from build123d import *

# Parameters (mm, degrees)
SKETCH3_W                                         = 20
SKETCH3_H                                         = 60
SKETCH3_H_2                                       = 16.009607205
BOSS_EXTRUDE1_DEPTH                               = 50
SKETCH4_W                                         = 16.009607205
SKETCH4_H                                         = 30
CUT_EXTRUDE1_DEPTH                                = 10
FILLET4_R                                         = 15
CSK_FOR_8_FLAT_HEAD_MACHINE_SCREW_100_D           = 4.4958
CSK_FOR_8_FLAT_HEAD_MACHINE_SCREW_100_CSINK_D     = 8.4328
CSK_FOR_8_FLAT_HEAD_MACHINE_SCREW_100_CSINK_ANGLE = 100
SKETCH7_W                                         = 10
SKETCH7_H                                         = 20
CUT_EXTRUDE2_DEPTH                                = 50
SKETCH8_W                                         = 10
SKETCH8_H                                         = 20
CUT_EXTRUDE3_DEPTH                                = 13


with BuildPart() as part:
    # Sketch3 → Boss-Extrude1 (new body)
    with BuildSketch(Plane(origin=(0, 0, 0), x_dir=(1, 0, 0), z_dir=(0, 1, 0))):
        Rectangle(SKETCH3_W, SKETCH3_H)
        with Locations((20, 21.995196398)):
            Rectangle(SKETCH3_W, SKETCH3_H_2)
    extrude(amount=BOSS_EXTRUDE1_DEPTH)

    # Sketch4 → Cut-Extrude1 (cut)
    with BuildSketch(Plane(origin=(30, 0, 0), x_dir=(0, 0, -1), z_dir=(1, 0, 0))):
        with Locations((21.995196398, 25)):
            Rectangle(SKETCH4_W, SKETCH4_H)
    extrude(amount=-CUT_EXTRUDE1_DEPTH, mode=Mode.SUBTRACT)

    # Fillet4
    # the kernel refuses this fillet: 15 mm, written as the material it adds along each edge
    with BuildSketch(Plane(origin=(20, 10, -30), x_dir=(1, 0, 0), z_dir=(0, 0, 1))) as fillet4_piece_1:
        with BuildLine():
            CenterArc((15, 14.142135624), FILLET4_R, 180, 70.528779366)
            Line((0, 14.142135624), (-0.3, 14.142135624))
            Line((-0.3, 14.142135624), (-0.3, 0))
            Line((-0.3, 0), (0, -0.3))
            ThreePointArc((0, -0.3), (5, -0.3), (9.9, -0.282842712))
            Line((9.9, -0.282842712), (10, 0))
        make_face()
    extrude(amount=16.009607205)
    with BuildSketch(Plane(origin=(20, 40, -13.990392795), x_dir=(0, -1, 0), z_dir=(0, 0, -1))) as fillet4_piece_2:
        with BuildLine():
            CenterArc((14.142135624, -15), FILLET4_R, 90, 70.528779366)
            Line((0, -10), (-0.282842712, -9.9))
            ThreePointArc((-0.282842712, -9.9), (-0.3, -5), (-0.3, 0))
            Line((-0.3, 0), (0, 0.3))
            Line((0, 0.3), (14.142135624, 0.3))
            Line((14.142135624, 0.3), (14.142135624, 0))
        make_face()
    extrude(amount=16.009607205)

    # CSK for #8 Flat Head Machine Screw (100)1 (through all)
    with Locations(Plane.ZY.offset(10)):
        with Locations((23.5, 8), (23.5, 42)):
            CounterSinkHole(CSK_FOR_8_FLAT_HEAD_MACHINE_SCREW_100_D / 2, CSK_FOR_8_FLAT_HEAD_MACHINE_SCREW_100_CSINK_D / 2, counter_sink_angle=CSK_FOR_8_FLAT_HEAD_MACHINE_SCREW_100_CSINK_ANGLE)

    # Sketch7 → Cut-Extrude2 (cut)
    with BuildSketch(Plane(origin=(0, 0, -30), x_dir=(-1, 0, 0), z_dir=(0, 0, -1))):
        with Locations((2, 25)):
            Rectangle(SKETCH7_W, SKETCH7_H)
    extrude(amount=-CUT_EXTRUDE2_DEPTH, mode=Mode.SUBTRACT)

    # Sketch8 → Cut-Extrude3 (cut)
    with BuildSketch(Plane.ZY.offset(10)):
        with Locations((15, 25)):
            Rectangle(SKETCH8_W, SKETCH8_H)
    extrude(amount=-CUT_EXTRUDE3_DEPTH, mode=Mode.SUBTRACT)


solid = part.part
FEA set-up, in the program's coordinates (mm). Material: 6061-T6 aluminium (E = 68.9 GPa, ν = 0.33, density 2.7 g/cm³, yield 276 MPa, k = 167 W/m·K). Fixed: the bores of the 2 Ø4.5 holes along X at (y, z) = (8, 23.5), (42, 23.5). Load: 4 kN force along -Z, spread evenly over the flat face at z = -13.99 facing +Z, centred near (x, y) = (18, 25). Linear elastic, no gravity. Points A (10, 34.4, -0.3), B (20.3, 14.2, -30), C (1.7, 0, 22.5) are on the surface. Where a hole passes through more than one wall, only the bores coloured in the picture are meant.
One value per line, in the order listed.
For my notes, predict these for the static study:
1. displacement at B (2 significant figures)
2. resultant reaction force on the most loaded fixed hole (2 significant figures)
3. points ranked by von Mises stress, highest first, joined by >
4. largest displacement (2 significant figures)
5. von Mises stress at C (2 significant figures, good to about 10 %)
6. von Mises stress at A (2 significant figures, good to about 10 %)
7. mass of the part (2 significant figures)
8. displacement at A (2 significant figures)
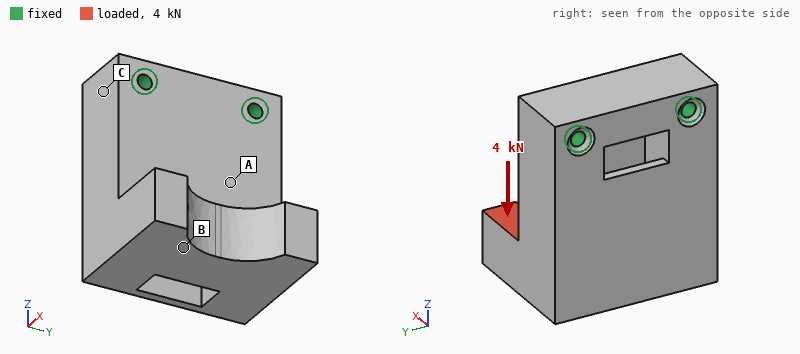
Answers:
79 µm
2.0 kN
A > C > B
94 µm
11 MPa
26 MPa
170 g
20 µm
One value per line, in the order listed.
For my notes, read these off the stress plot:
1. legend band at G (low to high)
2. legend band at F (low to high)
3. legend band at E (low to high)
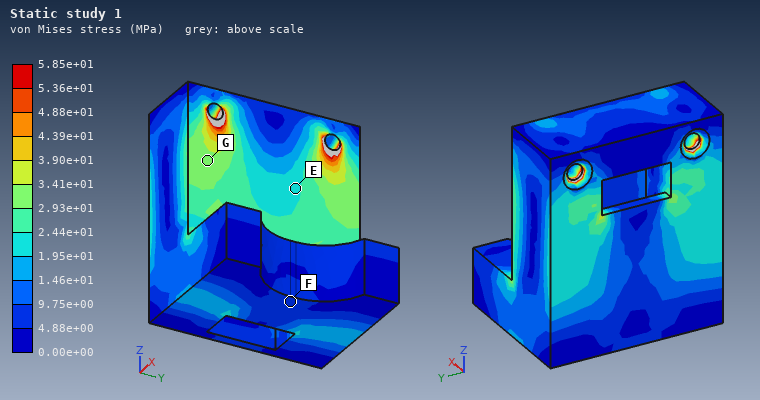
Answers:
2.93e+01 to 3.41e+01 MPa
4.88e+00 to 9.75e+00 MPa
1.95e+01 to 2.44e+01 MPa
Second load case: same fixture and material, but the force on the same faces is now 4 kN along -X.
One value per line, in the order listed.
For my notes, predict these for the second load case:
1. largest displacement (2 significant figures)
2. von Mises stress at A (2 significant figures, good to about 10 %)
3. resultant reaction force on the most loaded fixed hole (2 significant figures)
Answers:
0.10 mm
18 MPa
2.0 kN
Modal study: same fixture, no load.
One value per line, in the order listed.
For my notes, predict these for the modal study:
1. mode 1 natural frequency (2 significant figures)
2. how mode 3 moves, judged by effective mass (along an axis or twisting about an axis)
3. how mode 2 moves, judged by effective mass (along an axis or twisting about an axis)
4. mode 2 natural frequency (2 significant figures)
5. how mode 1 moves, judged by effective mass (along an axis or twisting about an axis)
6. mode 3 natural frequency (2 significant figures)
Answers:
3300 Hz
along Y
along Y
6100 Hz
along X
6900 Hz
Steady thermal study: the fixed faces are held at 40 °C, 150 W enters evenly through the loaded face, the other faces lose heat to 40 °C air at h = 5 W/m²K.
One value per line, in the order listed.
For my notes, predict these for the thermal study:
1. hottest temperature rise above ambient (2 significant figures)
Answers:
73 K
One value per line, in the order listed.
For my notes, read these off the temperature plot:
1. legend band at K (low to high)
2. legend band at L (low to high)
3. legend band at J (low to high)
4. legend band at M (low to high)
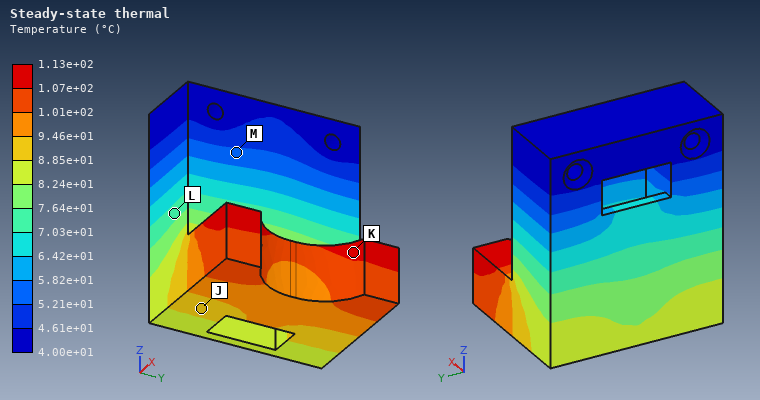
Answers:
1.07e+02 to 1.13e+02 °C
7.03e+01 to 7.64e+01 °C
8.85e+01 to 9.46e+01 °C
5.21e+01 to 5.82e+01 °C
